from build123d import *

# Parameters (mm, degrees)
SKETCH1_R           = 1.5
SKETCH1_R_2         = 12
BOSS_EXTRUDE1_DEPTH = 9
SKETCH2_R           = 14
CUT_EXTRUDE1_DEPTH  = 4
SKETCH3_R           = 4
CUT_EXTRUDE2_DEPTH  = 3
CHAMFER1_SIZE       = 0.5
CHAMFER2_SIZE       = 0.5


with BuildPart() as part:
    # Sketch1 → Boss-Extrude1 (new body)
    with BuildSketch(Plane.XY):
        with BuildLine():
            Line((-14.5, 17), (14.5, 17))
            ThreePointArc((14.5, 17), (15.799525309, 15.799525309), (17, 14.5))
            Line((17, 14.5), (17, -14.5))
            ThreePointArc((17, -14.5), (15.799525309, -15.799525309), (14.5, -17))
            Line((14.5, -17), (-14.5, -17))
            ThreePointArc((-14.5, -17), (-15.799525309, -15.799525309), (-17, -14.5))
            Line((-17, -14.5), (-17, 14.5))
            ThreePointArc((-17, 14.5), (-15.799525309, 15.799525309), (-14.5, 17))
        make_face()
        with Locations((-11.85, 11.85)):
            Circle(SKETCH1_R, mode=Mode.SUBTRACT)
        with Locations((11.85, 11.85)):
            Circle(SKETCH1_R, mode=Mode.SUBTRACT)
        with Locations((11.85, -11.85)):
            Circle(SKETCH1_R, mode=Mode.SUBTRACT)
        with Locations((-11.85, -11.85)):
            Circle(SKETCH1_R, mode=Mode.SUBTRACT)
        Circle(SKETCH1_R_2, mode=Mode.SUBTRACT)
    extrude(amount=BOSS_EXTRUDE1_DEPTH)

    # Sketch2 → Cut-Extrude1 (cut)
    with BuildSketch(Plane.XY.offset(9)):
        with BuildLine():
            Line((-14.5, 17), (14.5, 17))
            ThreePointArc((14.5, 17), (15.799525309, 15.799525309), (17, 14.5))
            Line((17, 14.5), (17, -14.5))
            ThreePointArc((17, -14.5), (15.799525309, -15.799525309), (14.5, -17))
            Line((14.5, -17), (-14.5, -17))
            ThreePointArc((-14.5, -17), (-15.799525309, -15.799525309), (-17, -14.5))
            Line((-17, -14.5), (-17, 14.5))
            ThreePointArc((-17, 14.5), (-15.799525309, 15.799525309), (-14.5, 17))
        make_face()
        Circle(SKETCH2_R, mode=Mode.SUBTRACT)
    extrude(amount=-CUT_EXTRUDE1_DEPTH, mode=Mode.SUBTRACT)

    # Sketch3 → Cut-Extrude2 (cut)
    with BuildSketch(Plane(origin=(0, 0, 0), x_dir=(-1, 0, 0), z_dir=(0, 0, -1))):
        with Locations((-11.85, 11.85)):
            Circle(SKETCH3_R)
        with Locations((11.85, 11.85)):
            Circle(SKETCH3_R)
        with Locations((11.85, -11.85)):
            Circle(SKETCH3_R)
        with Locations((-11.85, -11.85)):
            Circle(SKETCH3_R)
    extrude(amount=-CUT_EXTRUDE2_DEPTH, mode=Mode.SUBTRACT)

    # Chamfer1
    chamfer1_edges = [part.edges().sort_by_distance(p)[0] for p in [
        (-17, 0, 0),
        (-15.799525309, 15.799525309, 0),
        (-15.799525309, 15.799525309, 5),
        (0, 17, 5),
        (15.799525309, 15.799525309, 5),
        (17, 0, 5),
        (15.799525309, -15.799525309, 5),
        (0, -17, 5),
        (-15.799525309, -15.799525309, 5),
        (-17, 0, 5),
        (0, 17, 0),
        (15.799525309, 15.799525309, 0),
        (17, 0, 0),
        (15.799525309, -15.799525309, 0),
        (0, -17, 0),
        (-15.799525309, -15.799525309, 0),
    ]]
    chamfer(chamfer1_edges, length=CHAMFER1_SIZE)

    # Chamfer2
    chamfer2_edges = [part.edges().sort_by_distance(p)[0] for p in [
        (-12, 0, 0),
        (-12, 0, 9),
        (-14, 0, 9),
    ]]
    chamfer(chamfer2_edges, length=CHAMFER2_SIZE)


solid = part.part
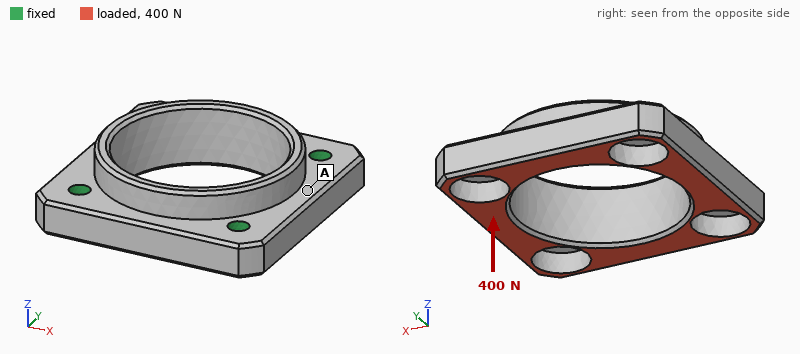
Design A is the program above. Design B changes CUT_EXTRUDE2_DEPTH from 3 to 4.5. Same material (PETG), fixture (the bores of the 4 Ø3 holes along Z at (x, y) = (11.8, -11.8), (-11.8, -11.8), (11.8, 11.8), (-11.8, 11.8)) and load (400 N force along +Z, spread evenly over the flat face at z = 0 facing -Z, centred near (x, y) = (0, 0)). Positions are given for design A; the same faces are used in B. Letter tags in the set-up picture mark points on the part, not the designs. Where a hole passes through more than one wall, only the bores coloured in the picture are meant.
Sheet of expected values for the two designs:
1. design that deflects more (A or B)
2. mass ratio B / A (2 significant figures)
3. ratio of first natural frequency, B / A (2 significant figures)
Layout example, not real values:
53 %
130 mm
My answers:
B
0.92
0.55
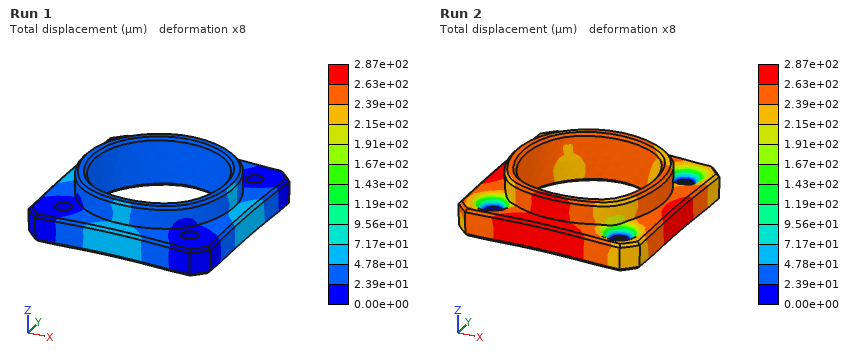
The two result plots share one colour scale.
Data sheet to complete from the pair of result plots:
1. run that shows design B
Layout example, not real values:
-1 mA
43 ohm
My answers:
Run 2
